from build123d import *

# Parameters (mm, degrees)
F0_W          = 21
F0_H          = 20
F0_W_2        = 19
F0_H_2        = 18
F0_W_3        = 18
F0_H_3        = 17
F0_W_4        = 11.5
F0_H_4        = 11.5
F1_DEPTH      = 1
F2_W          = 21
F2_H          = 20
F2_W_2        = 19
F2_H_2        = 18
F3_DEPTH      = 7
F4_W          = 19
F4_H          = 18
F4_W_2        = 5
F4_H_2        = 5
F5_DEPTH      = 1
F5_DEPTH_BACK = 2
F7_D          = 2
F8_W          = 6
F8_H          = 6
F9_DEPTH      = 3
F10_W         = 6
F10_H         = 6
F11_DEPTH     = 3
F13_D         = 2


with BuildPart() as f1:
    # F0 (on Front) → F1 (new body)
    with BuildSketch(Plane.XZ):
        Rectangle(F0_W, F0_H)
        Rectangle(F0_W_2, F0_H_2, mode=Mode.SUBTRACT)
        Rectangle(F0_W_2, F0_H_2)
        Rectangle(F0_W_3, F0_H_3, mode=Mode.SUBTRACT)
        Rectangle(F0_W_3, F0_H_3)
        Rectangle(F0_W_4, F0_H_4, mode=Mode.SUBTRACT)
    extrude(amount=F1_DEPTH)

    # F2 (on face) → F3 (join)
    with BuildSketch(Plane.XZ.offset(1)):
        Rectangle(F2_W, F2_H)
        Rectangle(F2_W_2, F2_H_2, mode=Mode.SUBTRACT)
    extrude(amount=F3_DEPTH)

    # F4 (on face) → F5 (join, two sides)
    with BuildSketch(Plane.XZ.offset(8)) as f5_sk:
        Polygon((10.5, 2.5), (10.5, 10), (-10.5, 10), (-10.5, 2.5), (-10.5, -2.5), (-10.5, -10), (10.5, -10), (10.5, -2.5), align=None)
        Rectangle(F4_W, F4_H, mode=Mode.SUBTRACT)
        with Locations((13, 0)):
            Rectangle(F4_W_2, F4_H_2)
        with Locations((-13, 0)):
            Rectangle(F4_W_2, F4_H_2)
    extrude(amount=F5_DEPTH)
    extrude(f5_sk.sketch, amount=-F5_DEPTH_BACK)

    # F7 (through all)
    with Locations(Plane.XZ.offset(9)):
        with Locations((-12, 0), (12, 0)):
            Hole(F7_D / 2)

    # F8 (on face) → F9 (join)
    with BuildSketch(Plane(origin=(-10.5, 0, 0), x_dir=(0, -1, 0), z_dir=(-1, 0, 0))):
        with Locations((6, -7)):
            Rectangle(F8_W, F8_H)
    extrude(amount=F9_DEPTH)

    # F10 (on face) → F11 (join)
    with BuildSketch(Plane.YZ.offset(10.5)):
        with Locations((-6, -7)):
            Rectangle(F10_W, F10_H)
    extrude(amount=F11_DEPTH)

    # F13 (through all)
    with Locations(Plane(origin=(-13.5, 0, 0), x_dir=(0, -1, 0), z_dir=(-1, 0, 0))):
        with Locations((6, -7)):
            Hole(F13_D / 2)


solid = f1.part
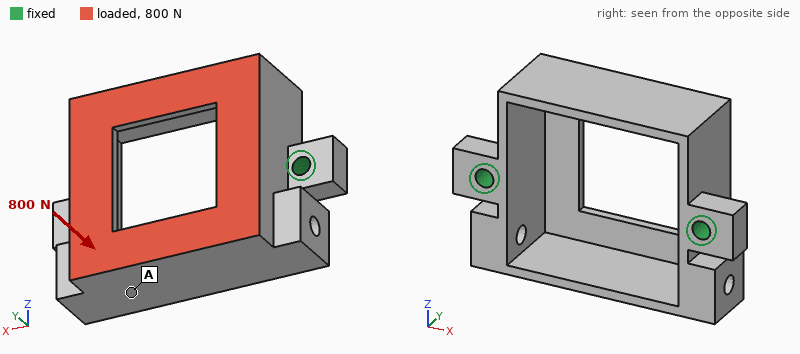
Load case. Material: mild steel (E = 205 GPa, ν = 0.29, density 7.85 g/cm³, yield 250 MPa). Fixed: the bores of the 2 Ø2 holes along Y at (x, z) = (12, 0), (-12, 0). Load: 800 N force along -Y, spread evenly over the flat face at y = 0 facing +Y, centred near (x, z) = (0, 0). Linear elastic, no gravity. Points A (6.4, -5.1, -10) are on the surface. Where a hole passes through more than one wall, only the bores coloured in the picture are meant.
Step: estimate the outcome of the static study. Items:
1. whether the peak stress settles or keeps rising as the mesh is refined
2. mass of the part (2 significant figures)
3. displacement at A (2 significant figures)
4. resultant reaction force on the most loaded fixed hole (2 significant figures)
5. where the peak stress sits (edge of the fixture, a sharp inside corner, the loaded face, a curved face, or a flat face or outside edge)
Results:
keeps rising
9.7 g
5.6 µm
410 N
edge of the fixture
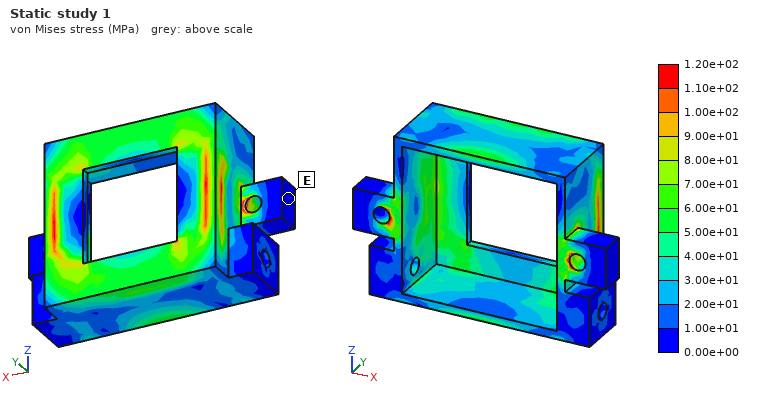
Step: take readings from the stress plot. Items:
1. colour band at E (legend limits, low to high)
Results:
0.00e+00 to 1.00e+01 MPa
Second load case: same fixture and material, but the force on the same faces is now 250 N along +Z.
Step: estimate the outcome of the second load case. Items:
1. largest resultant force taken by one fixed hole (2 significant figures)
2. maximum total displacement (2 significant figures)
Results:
130 N
12 µm
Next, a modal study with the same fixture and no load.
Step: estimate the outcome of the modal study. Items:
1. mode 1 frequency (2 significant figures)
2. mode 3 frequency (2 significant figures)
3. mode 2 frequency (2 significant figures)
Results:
8900 Hz
9700 Hz
9000 Hz
